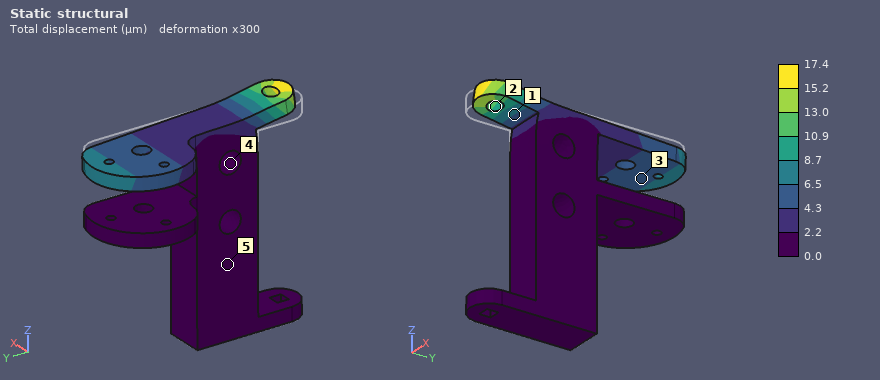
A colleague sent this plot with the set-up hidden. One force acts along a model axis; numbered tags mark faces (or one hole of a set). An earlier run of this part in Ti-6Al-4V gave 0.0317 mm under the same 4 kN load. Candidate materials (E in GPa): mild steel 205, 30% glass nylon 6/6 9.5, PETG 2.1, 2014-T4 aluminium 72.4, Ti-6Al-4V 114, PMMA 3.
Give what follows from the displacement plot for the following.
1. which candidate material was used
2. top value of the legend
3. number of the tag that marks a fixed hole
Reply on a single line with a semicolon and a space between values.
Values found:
mild steel; 17.4 µm; 4
